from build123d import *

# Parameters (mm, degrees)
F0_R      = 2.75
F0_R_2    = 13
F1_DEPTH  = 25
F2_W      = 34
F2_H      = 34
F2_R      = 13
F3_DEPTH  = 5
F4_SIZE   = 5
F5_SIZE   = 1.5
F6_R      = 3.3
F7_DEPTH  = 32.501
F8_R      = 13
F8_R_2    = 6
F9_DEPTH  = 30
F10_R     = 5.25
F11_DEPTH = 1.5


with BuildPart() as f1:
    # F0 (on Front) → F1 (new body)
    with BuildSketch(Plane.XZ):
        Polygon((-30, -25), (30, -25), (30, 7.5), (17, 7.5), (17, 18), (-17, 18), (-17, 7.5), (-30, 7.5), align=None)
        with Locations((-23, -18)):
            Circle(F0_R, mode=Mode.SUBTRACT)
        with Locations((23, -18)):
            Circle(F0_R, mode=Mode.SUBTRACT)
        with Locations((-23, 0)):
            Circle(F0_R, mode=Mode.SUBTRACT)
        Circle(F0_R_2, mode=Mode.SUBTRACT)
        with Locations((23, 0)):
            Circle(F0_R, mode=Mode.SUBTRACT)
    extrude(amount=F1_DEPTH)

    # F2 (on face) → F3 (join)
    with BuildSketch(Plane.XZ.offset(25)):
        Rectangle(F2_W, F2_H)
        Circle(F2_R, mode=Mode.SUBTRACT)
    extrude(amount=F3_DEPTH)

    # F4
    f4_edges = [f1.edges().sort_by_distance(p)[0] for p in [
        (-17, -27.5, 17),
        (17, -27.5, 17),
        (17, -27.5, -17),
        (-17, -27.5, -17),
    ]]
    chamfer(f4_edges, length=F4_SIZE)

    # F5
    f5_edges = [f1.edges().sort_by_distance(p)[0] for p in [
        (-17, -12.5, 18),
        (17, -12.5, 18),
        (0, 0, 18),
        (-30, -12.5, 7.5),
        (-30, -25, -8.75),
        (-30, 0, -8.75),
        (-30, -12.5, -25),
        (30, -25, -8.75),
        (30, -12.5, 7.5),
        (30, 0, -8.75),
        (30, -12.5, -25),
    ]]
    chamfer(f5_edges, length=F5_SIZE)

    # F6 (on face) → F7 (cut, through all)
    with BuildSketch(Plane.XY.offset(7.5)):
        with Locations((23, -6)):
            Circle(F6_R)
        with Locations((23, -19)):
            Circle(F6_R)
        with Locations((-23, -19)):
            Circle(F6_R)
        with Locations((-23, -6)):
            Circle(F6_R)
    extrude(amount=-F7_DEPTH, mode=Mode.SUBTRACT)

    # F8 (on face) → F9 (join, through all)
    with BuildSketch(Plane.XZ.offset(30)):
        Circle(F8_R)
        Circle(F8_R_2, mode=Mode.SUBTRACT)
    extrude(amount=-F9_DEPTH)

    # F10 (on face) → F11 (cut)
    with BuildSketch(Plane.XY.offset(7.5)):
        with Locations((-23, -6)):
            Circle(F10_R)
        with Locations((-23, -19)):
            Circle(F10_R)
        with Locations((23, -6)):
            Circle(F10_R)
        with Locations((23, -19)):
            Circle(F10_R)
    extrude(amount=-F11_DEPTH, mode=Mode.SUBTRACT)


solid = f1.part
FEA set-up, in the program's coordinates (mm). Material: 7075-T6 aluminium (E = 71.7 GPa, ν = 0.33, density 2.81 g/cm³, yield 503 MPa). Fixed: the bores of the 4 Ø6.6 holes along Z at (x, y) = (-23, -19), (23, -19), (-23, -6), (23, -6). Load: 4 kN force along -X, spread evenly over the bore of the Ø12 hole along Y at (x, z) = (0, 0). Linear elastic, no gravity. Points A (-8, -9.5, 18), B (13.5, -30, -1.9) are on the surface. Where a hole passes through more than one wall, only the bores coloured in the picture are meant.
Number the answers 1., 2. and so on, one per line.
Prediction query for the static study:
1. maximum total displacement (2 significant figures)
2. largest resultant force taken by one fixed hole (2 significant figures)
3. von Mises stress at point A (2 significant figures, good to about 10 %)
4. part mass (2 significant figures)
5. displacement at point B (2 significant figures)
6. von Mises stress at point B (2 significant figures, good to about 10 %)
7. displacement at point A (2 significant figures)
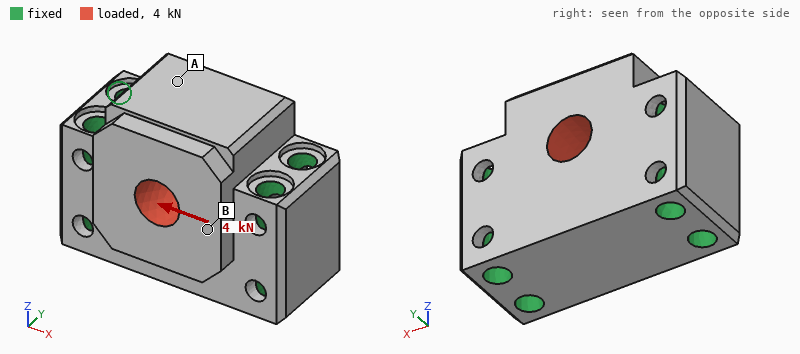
1. 1.4 µm
2. 1.1 kN
3. 0.97 MPa
4. 150 g
5. 0.82 µm
6. 2.5 MPa
7. 0.76 µm
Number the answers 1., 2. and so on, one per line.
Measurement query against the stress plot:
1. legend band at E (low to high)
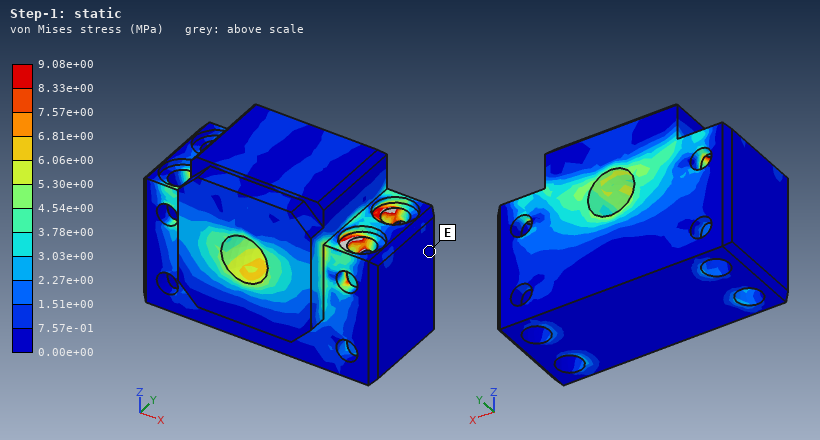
1. 0.00e+00 to 7.57e-01 MPa
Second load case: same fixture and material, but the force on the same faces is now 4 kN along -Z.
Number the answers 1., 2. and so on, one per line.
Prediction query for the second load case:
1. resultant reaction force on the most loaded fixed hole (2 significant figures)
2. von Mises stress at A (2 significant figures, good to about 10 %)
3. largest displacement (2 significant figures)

1. 1.2 kN
2. 2.2 MPa
3. 2.5 µm
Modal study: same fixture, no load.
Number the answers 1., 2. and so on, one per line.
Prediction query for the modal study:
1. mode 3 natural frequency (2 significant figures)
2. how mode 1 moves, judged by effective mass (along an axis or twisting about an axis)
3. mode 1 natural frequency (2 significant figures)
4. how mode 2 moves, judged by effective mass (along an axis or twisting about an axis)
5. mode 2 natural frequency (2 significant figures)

1. 31 kHz
2. along Y
3. 19 kHz
4. along Z
5. 29 kHz
